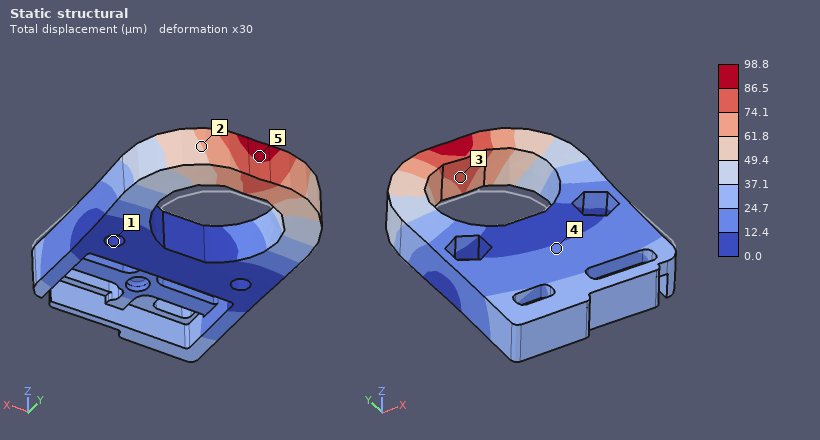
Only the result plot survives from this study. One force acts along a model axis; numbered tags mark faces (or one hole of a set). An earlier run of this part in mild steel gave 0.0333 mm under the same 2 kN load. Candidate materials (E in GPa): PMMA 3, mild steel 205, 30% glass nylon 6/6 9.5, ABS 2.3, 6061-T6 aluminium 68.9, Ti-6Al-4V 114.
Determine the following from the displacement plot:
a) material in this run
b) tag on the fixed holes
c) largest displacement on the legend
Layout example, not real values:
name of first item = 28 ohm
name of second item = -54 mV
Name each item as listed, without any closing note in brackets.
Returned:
material in this run = 6061-T6 aluminium
tag on the fixed holes = 1
largest displacement on the legend = 98.8 µm
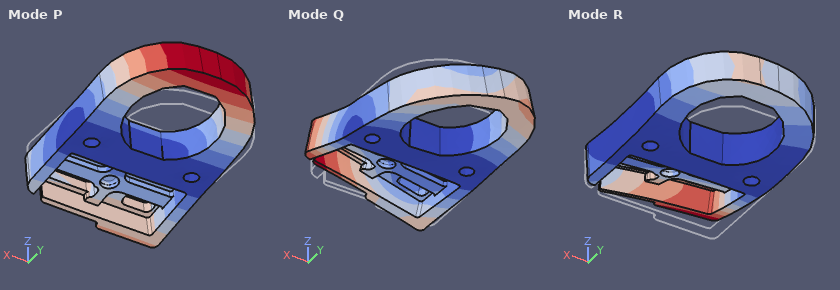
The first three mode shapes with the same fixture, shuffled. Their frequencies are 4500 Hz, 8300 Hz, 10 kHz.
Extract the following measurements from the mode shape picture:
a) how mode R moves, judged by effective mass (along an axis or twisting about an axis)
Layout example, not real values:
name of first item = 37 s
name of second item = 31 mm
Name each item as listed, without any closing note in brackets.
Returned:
how mode R moves, judged by effective mass = along Z
